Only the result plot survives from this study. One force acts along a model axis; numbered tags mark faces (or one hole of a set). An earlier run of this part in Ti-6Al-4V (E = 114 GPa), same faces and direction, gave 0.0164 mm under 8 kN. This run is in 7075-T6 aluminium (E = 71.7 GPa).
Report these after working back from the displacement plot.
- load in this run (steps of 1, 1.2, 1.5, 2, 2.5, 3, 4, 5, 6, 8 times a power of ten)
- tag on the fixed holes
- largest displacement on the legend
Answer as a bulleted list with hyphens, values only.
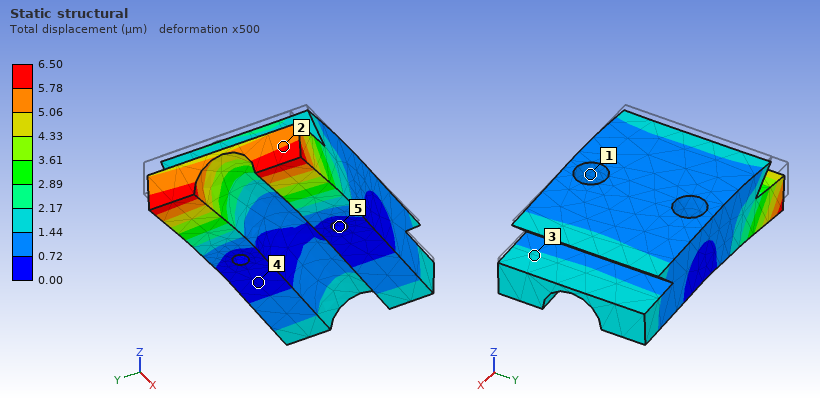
- 2 kN
- 5
- 6.50 µm
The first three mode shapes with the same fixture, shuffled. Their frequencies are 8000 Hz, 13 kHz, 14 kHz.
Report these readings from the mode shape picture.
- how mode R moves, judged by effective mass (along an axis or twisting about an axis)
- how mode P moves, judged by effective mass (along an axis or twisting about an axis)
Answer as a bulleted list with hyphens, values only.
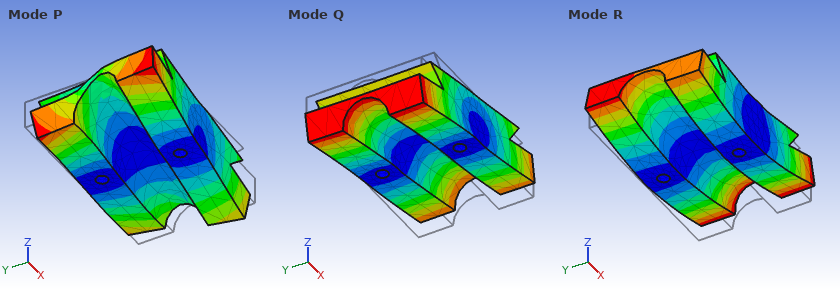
- along Z
- twisting about Z
